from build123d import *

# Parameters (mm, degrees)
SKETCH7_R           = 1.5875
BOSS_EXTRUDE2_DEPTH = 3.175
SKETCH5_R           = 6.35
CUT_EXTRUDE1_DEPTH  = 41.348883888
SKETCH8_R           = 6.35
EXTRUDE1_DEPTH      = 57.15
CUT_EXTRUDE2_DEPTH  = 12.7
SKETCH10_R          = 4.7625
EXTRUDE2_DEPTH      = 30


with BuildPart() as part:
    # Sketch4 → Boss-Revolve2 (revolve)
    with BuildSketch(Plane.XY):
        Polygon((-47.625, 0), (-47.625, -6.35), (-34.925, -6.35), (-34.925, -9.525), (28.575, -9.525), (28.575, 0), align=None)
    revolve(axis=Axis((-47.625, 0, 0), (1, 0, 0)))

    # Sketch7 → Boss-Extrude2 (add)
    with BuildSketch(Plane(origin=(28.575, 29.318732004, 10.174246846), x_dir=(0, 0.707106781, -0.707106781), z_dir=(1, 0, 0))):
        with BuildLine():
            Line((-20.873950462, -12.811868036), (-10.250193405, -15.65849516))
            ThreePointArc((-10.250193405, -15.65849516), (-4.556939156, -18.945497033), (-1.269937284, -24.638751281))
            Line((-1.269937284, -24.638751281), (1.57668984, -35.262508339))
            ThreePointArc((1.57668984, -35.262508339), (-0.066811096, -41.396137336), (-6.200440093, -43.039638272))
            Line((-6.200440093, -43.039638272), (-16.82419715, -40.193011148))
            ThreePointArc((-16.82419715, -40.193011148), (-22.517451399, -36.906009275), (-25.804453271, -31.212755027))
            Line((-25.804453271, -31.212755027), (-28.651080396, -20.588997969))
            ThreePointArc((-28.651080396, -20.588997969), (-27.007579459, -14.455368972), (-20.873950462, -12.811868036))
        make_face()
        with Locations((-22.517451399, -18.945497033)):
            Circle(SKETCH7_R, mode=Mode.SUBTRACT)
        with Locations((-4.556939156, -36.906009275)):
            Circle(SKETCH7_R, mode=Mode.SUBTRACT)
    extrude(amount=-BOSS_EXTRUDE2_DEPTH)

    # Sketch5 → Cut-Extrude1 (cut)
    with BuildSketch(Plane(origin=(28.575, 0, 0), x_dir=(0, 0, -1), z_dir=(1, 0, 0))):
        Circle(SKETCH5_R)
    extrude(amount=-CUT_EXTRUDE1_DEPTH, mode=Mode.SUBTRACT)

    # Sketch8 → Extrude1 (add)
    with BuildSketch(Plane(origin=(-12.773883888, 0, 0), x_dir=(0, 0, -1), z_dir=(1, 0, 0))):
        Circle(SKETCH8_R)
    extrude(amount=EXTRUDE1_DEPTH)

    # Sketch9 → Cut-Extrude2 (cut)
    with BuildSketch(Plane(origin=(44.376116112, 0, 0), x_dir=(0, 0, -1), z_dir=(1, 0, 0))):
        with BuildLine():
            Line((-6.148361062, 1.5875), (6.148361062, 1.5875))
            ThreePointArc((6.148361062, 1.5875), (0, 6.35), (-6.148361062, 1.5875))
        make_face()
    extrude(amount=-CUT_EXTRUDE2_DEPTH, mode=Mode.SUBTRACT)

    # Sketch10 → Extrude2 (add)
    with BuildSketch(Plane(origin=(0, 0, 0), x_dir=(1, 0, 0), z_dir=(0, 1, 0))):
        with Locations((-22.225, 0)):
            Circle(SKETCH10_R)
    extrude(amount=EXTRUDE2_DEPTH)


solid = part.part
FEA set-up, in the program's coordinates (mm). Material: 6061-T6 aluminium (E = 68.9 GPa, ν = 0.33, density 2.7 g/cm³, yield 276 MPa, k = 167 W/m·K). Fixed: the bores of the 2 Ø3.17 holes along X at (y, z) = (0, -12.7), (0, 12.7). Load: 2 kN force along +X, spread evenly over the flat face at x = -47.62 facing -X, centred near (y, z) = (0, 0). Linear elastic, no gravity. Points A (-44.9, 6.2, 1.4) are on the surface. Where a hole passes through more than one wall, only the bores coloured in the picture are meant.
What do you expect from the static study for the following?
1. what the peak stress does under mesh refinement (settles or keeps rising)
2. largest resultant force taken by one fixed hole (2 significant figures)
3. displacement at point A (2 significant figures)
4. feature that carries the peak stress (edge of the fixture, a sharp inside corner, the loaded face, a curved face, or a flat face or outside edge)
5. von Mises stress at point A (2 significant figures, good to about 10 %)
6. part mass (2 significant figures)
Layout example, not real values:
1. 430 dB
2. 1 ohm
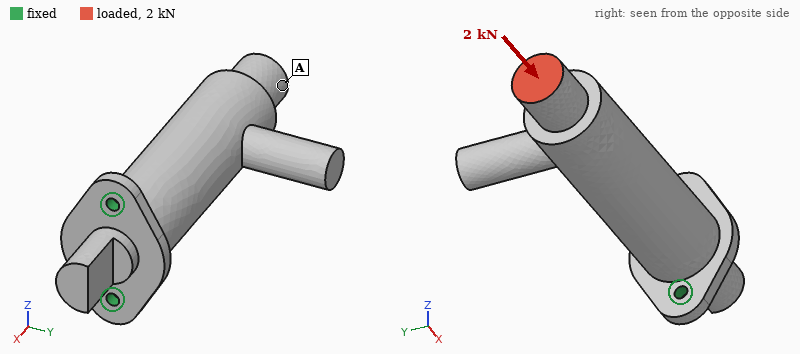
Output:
1. keeps rising
2. 1.1 kN
3. 19 µm
4. edge of the fixture
5. 16 MPa
6. 64 g
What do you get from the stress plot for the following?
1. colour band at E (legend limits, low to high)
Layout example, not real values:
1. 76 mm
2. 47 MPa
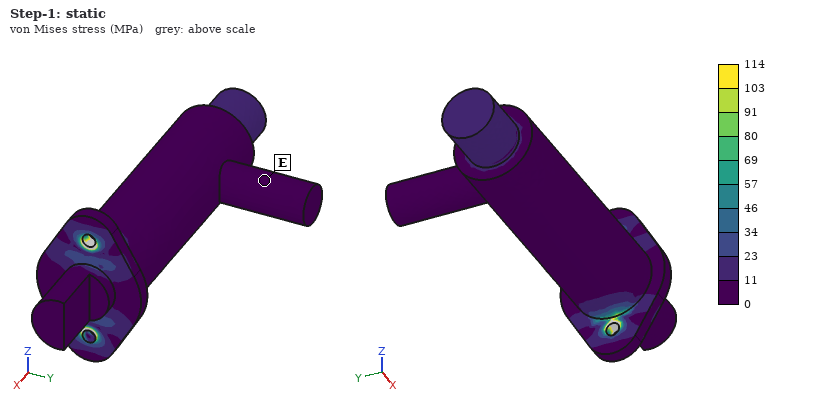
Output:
1. 0 to 11 MPa
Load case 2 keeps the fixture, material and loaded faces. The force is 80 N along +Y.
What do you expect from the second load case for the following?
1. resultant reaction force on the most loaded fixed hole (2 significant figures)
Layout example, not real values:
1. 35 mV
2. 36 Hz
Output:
1. 40 N
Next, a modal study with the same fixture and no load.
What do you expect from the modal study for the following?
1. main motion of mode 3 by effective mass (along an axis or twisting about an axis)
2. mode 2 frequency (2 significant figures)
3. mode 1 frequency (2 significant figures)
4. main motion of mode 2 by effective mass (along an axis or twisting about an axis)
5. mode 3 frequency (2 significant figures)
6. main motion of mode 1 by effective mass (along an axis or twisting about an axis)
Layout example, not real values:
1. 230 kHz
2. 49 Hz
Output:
1. twisting about X
2. 1900 Hz
3. 710 Hz
4. along Z
5. 6800 Hz
6. along Y
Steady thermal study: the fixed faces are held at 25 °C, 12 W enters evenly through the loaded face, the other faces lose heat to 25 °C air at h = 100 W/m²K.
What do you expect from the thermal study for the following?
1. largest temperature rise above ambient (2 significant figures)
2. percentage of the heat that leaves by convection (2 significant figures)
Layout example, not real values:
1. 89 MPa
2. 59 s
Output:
1. 21 K
2. 42 %
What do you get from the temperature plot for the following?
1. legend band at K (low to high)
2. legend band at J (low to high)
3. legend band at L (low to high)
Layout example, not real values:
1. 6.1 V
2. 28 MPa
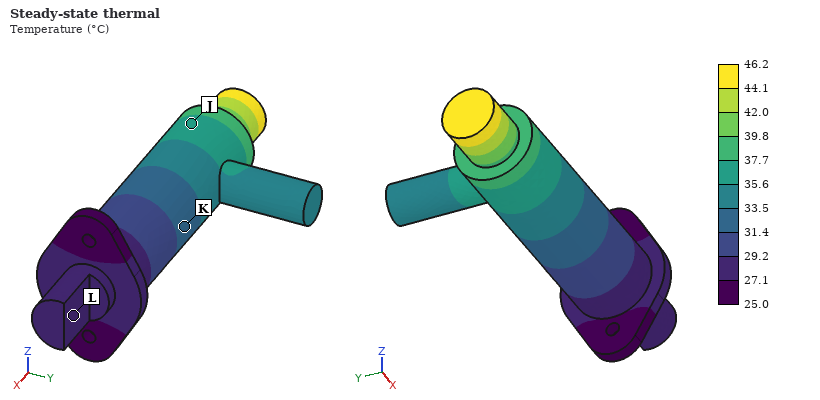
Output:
1. 31.4 to 33.5 °C
2. 35.6 to 37.7 °C
3. 27.1 to 29.2 °C
